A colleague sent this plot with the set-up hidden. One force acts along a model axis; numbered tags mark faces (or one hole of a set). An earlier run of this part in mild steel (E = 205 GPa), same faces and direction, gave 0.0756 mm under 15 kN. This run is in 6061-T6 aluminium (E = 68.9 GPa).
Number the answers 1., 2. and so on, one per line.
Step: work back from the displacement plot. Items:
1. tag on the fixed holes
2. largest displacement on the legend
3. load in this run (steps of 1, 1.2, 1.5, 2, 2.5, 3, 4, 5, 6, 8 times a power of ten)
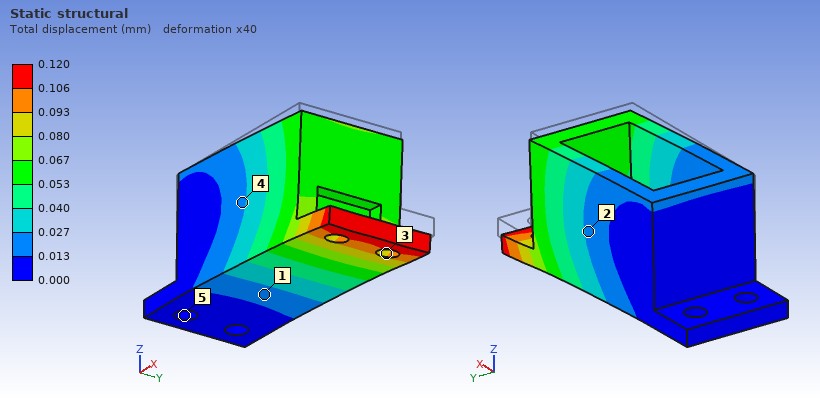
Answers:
1. 5
2. 0.120 mm
3. 8 kN
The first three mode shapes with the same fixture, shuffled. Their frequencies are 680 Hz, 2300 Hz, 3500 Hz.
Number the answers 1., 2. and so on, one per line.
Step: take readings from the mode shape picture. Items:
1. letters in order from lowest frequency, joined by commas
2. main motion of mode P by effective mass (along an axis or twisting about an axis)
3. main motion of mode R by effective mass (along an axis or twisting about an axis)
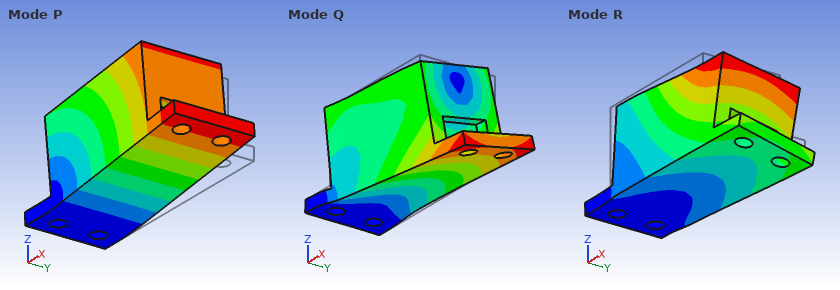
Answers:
1. P, R, Q
2. along Z
3. along Y
